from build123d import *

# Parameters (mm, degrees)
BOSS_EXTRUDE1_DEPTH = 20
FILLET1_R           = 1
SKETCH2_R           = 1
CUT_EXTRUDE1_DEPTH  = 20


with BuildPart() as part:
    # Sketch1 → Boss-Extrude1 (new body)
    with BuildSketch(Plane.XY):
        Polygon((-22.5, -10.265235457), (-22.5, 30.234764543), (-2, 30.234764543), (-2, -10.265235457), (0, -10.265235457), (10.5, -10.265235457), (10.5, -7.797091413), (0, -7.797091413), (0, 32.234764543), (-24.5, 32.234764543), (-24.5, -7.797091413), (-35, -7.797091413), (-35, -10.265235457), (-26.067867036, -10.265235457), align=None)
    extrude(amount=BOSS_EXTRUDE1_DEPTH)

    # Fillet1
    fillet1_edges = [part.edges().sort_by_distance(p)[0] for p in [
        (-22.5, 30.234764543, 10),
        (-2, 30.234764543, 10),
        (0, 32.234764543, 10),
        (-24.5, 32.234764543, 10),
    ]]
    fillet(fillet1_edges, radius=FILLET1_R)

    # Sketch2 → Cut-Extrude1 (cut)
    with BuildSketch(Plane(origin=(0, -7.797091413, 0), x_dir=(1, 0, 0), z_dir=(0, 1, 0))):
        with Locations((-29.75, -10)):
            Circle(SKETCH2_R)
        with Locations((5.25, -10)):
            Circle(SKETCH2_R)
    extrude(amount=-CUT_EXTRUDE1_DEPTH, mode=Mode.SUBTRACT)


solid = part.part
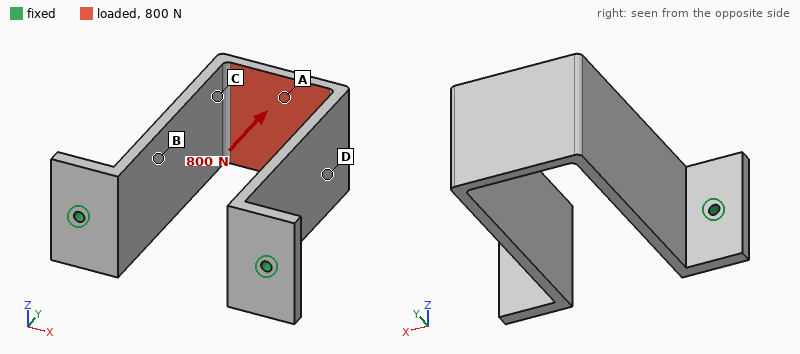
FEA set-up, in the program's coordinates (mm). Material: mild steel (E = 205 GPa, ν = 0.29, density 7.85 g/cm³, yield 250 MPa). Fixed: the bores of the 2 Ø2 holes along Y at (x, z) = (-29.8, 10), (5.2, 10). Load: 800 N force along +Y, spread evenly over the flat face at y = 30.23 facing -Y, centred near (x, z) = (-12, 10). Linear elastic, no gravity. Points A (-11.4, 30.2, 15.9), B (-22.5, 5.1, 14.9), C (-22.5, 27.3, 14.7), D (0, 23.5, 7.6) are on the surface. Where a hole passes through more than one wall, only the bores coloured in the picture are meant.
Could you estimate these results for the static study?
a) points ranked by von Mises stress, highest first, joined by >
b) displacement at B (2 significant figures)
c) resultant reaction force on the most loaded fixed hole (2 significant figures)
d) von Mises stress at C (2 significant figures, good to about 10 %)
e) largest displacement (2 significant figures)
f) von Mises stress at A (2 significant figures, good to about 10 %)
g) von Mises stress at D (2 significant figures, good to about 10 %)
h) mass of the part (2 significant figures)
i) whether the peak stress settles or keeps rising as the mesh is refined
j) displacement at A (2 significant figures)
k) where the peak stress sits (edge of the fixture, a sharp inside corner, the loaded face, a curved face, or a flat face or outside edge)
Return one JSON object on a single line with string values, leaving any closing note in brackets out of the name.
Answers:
{"points ranked by von Mises stress, highest first, joined by >": "A > C > D > B", "displacement at B": "8.2 µm", "resultant reaction force on the most loaded fixed hole": "400 N", "von Mises stress at C": "71 MPa", "largest displacement": "38 µm", "von Mises stress at A": "110 MPa", "von Mises stress at D": "39 MPa", "mass of the part": "41 g", "whether the peak stress settles or keeps rising as the mesh is refined": "keeps rising", "displacement at A": "35 µm", "where the peak stress sits": "edge of the fixture"}
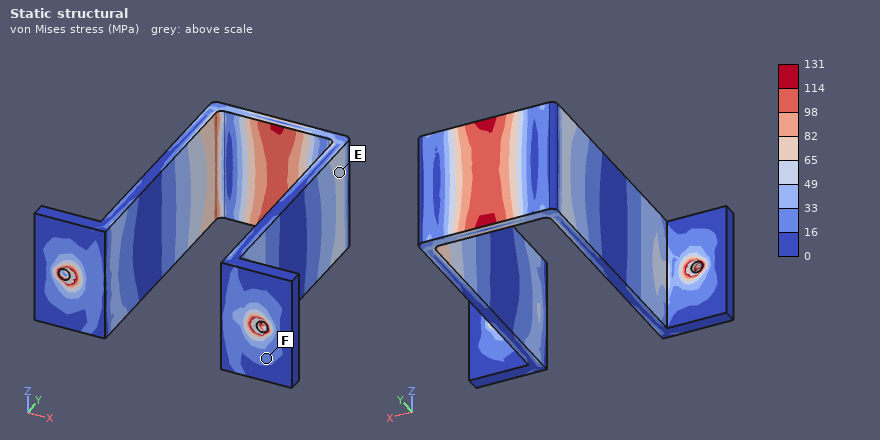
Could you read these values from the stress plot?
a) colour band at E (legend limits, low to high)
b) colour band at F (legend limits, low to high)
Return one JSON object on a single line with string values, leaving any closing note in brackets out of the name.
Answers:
{"colour band at E": "49 to 65 MPa", "colour band at F": "16 to 33 MPa"}
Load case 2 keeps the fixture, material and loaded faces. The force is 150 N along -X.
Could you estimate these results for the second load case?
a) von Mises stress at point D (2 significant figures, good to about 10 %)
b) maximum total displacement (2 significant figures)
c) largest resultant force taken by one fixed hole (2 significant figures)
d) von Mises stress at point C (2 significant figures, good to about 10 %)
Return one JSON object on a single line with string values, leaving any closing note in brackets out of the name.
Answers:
{"von Mises stress at point D": "60 MPa", "maximum total displacement": "0.19 mm", "largest resultant force taken by one fixed hole": "150 N", "von Mises stress at point C": "89 MPa"}
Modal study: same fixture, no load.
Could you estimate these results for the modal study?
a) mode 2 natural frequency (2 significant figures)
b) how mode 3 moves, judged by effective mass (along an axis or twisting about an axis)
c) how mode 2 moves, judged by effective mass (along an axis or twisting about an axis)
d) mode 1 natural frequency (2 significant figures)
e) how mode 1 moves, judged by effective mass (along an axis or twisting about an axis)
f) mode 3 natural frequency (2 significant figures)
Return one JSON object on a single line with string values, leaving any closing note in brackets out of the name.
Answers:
{"mode 2 natural frequency": "1300 Hz", "how mode 3 moves, judged by effective mass": "twisting about Y", "how mode 2 moves, judged by effective mass": "along Z", "mode 1 natural frequency": "1100 Hz", "how mode 1 moves, judged by effective mass": "along X", "mode 3 natural frequency": "2400 Hz"}
